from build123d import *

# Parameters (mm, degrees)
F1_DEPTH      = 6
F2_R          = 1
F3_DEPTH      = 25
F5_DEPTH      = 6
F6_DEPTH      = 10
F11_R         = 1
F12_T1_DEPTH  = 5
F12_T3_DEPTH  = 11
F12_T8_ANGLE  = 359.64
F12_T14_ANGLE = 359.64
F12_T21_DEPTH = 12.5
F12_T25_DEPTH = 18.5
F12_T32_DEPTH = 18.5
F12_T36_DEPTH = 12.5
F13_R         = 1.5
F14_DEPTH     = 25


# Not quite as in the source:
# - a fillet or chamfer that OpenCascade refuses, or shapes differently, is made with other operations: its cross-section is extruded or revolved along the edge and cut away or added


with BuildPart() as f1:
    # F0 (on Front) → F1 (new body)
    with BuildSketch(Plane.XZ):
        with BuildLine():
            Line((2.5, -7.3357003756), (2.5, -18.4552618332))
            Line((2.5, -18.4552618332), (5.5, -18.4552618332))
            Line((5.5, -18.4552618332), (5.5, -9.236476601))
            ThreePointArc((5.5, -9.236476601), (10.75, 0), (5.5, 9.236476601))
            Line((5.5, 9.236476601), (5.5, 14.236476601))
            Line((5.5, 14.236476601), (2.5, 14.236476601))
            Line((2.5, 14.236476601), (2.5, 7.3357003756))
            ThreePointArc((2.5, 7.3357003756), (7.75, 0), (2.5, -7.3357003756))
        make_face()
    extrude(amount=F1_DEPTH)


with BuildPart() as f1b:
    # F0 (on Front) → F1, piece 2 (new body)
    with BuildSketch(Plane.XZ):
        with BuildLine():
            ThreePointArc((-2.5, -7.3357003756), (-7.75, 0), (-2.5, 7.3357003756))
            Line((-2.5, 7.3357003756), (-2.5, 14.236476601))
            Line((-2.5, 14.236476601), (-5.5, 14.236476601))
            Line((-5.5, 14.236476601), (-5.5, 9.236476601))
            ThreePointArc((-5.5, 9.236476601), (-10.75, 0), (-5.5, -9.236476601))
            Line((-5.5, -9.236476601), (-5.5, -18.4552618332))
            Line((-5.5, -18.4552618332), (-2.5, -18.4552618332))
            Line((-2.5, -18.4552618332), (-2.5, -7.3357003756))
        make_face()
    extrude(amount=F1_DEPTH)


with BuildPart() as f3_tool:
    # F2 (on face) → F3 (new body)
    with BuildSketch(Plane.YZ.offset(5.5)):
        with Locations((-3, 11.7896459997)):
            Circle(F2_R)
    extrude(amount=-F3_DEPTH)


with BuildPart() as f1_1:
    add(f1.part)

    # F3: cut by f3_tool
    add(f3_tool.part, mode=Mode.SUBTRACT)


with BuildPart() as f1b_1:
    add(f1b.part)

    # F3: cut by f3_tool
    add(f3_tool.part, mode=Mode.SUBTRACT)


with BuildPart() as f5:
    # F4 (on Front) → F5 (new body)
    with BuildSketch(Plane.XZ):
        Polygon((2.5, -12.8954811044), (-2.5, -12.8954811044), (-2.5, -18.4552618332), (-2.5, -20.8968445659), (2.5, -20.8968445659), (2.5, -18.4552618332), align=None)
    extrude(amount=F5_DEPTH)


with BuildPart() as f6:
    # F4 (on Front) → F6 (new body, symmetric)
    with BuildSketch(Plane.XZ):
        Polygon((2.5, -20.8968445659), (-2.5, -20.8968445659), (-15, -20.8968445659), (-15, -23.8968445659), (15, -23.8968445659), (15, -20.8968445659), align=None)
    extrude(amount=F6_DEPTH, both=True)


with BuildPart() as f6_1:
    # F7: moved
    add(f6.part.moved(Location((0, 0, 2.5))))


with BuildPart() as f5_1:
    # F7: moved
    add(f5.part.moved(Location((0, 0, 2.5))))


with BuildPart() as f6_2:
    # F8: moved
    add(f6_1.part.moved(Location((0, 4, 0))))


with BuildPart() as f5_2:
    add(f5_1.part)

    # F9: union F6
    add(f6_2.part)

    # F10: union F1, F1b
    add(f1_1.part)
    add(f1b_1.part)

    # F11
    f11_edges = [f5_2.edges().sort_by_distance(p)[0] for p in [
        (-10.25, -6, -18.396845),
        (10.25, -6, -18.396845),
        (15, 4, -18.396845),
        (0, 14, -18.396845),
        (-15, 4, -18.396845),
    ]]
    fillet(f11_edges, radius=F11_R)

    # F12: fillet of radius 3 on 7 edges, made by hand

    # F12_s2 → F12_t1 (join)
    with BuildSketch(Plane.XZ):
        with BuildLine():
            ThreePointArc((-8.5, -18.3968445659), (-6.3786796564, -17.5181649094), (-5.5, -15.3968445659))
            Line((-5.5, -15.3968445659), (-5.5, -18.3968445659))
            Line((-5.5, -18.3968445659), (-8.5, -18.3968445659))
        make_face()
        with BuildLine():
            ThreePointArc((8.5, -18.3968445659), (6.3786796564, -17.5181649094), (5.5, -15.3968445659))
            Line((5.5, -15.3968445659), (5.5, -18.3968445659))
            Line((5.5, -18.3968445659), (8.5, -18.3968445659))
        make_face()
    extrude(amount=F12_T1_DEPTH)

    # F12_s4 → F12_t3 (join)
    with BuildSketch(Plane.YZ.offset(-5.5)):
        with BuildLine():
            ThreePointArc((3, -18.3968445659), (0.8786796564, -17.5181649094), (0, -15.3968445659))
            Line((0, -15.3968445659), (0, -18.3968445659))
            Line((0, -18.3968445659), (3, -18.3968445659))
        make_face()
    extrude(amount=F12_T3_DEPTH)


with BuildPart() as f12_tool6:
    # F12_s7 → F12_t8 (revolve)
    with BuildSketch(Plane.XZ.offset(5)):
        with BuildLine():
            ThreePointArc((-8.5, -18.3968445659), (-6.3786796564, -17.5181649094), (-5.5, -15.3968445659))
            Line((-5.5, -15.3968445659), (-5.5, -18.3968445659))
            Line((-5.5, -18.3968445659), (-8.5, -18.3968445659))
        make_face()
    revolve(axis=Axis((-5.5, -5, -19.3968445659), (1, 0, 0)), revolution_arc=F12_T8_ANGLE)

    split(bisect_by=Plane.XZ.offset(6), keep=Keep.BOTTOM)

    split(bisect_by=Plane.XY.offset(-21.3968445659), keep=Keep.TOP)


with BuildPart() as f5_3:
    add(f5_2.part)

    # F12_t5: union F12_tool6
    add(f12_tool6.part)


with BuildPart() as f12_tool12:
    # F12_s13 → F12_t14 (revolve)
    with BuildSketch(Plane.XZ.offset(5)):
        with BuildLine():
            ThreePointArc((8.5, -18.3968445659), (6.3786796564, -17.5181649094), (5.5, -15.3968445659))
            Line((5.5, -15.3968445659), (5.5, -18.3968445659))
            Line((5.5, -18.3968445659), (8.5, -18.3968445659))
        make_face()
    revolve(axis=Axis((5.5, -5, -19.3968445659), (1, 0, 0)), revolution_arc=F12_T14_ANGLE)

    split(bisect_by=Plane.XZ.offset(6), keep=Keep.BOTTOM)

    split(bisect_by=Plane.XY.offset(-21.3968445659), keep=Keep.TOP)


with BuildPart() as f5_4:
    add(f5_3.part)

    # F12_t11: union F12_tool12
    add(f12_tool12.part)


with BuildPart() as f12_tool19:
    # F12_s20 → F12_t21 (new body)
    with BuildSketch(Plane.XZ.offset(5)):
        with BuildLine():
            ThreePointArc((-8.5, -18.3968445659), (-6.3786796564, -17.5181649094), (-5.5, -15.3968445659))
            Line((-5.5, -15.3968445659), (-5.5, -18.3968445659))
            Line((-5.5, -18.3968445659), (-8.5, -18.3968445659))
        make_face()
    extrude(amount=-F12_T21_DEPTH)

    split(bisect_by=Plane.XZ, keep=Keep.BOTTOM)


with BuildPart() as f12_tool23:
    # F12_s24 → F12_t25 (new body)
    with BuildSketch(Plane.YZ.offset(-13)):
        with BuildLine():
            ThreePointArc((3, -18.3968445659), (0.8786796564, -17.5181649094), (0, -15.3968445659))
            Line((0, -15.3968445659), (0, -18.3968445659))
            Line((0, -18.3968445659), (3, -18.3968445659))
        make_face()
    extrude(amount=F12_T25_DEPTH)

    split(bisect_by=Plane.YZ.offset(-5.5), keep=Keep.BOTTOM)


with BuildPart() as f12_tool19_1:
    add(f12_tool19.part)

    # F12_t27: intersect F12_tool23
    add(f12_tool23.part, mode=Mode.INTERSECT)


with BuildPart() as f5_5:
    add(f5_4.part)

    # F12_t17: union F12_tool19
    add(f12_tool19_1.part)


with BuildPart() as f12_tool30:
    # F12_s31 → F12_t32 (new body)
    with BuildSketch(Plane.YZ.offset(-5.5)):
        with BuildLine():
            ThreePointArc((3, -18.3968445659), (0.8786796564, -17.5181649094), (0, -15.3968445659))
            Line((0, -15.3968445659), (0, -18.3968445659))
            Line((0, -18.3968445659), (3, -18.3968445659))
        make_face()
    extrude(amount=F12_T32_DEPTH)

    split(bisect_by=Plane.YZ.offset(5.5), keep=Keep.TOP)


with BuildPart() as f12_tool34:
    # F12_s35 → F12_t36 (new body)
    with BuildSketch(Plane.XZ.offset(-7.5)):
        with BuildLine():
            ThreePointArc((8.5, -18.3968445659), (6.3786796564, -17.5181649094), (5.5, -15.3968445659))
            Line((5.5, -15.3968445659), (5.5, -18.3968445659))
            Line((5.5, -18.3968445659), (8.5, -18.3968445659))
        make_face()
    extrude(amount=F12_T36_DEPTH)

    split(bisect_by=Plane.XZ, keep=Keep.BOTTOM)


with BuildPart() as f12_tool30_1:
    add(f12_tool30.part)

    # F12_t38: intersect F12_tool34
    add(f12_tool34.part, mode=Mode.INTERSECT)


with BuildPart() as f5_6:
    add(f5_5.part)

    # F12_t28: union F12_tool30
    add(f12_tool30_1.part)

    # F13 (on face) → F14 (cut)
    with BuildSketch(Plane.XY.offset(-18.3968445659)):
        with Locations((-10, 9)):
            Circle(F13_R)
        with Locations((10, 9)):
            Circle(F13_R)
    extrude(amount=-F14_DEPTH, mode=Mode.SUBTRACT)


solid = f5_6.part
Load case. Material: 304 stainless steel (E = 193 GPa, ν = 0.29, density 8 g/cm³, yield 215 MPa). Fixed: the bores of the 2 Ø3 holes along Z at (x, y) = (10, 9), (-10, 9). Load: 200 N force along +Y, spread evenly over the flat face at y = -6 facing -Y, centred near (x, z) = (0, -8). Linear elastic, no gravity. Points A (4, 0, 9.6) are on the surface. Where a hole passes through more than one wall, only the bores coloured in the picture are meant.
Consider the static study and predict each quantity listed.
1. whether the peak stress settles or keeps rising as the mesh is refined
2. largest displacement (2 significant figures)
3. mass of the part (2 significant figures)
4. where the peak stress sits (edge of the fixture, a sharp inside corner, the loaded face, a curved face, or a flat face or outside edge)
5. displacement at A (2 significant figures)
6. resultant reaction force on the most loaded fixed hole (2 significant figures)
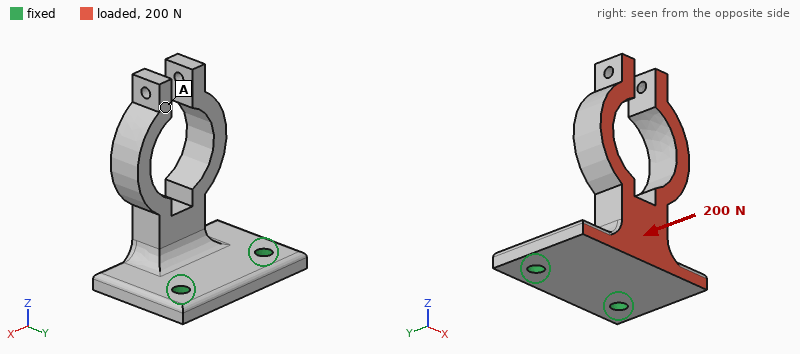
keeps rising
99 µm
27 g
edge of the fixture
81 µm
110 N
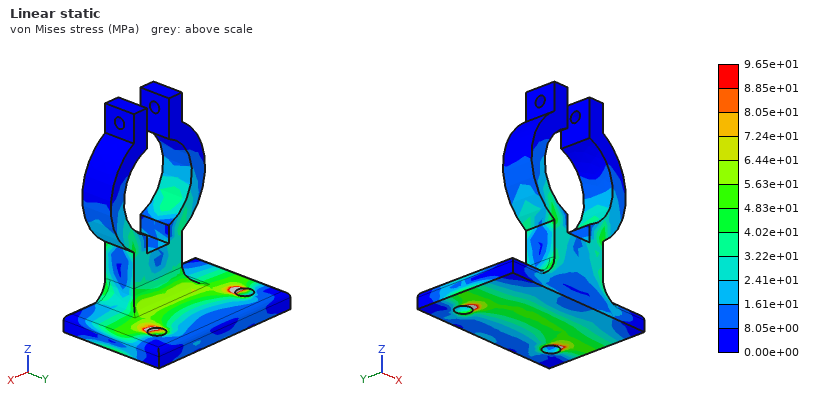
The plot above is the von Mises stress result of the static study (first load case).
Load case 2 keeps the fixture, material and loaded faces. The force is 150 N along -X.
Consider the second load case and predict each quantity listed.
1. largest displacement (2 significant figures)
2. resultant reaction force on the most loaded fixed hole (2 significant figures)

54 µm
160 N
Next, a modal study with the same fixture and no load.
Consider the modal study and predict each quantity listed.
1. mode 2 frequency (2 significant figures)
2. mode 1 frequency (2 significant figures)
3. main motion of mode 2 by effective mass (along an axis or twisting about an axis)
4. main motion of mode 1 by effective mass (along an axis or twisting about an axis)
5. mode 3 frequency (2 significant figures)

2700 Hz
2200 Hz
along X
along Y
3100 Hz
